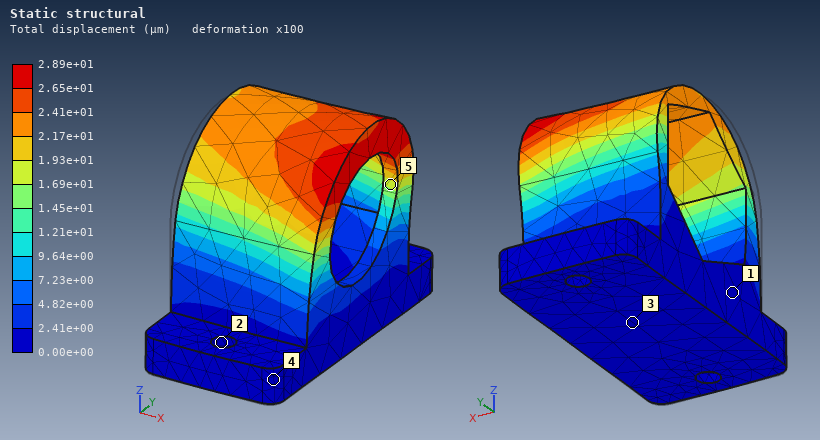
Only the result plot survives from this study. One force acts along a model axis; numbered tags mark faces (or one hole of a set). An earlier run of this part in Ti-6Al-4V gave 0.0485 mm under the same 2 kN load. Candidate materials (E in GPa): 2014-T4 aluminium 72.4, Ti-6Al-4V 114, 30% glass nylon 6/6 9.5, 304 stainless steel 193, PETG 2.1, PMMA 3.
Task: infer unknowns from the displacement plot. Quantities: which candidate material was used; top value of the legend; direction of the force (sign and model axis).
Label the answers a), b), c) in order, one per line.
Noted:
a) 304 stainless steel
b) 2.89e+01 µm
c) +Y
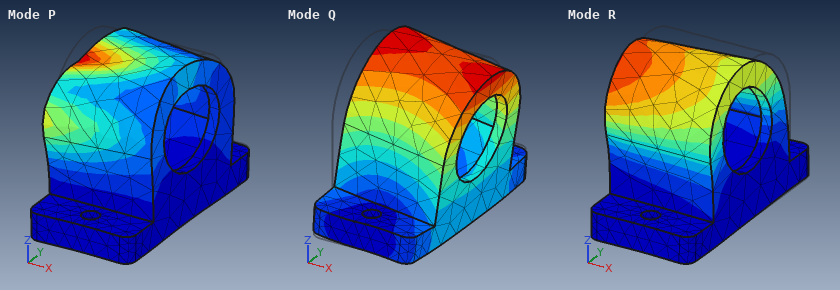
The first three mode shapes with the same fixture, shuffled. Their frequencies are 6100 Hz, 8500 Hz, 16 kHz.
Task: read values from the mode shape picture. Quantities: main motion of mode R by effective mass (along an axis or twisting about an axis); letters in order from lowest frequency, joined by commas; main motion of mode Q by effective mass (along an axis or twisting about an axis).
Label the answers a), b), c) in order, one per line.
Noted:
a) along Y
b) Q, R, P
c) along X
